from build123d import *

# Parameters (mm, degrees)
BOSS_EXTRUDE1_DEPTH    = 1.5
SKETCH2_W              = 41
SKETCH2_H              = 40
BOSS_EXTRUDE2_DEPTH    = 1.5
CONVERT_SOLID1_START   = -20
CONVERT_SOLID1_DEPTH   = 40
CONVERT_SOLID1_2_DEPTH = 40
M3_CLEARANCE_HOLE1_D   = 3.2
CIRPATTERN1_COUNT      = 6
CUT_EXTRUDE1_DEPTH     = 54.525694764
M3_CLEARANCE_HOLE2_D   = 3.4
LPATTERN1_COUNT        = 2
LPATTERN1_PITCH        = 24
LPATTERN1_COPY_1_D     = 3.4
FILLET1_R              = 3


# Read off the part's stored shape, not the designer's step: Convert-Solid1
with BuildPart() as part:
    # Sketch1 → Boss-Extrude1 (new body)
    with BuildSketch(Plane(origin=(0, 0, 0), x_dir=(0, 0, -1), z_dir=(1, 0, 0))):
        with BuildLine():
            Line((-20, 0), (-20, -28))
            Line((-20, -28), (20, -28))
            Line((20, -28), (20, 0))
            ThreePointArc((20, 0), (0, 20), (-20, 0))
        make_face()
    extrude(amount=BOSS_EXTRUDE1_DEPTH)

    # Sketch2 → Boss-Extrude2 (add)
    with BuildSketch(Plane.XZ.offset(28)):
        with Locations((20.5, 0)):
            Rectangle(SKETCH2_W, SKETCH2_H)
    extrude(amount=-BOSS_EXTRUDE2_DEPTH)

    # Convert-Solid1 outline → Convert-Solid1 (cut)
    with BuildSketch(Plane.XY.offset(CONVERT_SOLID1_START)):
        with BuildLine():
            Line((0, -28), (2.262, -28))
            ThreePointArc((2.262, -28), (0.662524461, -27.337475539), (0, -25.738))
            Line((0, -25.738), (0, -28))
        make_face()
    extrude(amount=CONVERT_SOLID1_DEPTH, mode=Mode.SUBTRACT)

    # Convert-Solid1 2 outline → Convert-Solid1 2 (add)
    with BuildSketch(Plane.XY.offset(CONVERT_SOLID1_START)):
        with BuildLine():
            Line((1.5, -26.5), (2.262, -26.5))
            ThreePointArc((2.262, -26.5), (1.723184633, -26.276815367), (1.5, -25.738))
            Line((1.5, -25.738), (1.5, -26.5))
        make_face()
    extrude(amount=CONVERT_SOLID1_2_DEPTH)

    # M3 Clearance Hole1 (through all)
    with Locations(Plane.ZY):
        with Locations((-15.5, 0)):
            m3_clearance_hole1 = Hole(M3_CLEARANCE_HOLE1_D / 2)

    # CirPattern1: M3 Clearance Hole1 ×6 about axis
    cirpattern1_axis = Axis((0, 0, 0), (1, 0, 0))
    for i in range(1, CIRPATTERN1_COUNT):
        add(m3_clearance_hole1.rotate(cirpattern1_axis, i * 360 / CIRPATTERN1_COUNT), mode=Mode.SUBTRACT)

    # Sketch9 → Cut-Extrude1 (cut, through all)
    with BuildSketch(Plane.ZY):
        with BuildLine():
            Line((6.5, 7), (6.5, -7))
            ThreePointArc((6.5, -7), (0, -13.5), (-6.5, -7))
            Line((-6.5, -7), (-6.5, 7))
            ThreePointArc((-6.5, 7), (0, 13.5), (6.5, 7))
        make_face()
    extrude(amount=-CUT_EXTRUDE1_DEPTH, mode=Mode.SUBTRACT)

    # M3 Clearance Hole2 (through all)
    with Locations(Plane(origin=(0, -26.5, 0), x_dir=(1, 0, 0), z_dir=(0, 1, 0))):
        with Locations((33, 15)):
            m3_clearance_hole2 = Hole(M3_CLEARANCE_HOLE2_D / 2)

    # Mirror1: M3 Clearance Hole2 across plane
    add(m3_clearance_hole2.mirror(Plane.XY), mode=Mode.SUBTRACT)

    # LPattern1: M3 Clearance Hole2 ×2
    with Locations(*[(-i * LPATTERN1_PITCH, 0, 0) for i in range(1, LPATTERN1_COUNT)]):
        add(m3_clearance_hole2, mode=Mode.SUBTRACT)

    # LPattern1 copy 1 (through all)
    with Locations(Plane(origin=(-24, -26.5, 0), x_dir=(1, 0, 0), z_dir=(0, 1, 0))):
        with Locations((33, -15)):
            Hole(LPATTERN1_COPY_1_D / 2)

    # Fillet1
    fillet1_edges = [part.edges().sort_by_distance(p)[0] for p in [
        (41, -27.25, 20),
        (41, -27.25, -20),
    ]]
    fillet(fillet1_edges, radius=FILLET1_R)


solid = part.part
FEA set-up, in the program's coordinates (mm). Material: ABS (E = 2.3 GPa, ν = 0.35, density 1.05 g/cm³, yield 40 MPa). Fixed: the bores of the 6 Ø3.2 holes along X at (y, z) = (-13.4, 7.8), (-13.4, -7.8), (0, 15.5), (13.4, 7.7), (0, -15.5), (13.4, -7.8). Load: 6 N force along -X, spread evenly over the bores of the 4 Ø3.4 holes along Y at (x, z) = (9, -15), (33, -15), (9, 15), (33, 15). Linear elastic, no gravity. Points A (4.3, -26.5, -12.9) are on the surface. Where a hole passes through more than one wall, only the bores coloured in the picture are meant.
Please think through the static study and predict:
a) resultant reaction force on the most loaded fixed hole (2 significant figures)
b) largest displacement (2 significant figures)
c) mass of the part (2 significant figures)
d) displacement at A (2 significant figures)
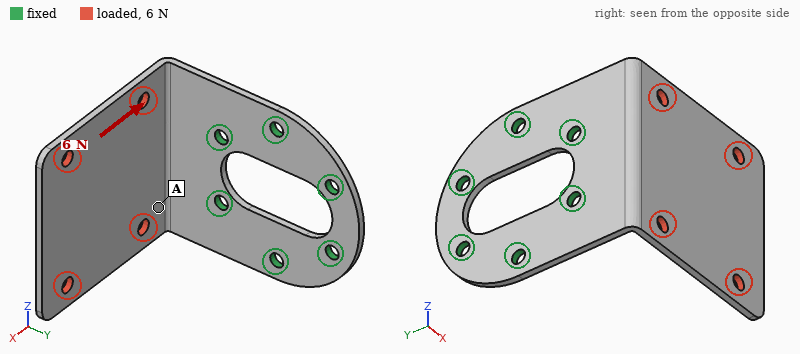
3.7 N
0.86 mm
4.6 g
0.20 mm
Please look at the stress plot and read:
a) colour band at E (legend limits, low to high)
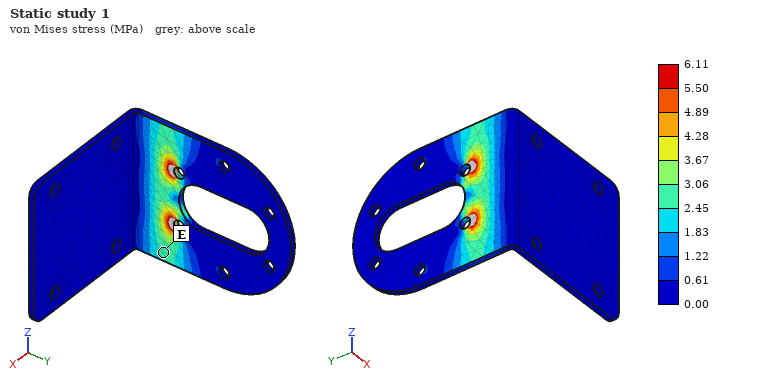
2.45 to 3.06 MPa
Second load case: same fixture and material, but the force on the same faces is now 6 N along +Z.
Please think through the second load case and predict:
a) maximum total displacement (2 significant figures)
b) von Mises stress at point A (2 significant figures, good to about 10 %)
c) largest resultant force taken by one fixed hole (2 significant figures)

0.74 mm
2.6 MPa
7.2 N
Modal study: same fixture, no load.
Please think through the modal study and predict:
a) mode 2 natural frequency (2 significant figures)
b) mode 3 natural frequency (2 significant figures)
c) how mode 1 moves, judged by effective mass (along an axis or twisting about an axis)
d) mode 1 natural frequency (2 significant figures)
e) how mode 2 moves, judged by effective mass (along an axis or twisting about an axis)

320 Hz
540 Hz
along Y
150 Hz
along Z
